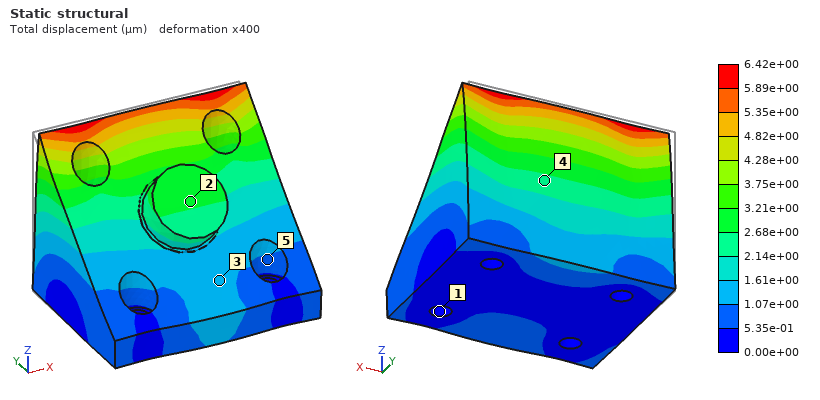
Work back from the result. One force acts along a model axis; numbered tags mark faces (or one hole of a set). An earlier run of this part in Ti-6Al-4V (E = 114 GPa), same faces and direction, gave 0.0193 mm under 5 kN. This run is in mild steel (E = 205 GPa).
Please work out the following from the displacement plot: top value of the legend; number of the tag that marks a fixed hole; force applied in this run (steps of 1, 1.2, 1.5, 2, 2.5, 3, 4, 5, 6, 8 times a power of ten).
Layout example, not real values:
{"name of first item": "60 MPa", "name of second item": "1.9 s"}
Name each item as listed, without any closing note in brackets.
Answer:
{"top value of the legend": "6.42e+00 µm", "number of the tag that marks a fixed hole": "1", "force applied in this run": "3 kN"}
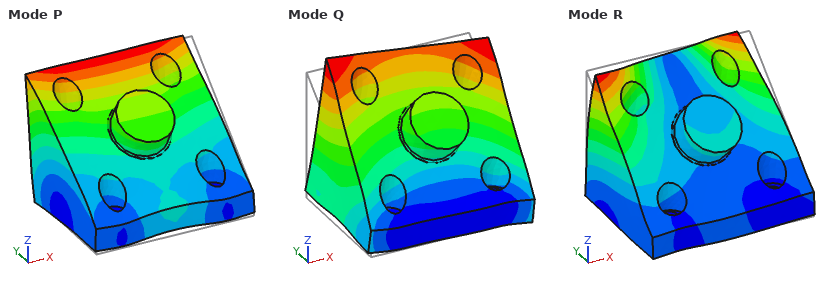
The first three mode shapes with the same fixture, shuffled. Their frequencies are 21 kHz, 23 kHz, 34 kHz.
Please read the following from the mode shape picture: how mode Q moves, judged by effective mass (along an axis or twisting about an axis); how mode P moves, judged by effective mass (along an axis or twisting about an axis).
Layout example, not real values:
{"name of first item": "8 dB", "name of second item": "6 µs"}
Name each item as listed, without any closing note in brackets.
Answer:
{"how mode Q moves, judged by effective mass": "along X", "how mode P moves, judged by effective mass": "along Y"}
